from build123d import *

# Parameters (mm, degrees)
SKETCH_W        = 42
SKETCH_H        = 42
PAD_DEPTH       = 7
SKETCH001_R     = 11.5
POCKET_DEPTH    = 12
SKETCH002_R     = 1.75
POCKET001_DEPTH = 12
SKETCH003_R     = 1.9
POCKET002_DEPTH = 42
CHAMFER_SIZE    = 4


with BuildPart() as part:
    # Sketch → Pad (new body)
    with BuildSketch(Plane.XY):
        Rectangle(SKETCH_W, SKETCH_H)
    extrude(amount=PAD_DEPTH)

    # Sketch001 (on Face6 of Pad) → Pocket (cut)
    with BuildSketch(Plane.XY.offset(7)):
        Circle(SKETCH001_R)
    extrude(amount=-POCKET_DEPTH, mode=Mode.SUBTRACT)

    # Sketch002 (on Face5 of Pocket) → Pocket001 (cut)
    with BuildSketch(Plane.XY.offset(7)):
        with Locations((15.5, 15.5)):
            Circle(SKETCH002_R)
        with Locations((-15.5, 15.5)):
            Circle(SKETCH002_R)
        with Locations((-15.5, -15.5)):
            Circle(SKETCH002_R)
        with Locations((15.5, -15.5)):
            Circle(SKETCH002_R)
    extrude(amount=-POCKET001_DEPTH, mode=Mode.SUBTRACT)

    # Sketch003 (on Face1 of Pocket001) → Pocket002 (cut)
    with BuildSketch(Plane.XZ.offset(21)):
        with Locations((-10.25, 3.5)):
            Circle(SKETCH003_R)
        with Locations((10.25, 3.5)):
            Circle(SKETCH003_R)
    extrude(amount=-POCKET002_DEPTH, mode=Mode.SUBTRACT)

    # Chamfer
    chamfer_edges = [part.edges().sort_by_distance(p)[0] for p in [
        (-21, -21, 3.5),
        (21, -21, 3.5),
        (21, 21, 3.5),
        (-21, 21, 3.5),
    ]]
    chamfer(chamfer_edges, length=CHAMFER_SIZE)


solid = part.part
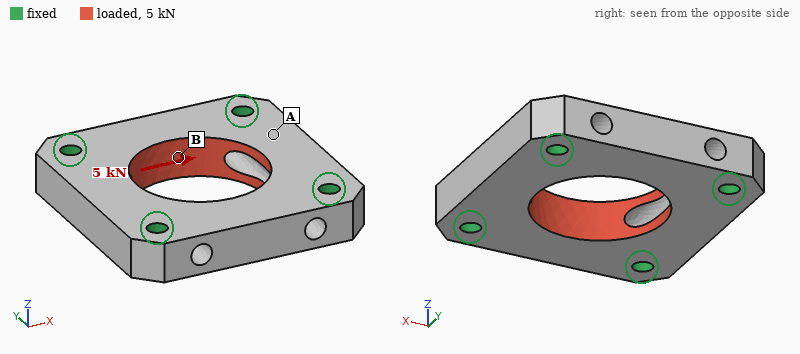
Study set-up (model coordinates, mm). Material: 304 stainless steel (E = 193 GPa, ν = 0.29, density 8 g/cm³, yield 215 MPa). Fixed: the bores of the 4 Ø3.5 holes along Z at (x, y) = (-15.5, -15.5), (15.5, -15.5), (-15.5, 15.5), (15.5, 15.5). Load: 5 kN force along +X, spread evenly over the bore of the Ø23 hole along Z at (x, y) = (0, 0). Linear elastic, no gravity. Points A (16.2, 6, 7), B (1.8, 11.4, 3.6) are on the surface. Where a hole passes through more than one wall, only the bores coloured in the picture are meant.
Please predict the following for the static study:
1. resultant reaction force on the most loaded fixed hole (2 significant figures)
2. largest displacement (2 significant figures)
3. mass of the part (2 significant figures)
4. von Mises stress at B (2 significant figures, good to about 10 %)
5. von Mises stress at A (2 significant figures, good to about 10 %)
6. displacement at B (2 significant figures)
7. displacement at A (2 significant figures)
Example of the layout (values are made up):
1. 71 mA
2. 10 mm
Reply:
1. 1.3 kN
2. 2.9 µm
3. 66 g
4. 22 MPa
5. 10.0 MPa
6. 1.6 µm
7. 1.6 µm
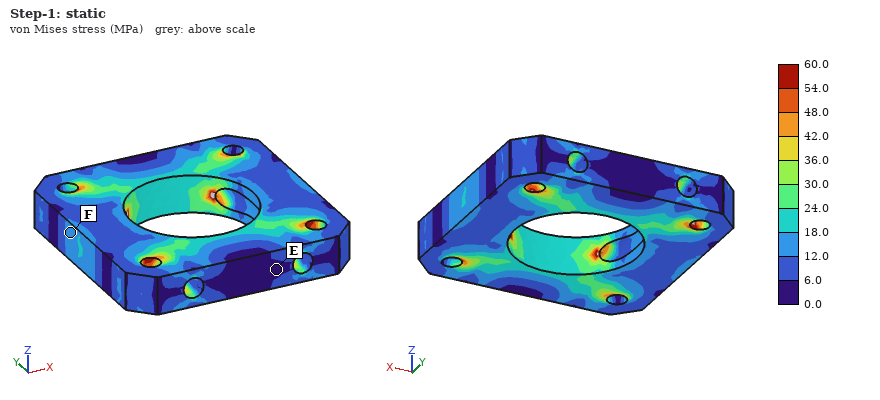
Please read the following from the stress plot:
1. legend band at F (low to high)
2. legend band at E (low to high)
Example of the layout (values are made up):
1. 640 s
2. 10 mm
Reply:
1. 12.0 to 18.0 MPa
2. 0.0 to 6.0 MPa
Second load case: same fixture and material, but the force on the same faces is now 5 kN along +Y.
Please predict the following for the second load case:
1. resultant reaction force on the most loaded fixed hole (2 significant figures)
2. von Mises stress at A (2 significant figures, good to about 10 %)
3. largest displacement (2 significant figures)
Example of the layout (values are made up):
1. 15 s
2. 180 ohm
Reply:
1. 1.3 kN
2. 13 MPa
3. 3.6 µm
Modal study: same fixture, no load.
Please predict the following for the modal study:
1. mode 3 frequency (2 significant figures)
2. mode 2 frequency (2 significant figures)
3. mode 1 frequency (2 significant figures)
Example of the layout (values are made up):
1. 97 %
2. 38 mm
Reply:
1. 27 kHz
2. 24 kHz
3. 24 kHz
